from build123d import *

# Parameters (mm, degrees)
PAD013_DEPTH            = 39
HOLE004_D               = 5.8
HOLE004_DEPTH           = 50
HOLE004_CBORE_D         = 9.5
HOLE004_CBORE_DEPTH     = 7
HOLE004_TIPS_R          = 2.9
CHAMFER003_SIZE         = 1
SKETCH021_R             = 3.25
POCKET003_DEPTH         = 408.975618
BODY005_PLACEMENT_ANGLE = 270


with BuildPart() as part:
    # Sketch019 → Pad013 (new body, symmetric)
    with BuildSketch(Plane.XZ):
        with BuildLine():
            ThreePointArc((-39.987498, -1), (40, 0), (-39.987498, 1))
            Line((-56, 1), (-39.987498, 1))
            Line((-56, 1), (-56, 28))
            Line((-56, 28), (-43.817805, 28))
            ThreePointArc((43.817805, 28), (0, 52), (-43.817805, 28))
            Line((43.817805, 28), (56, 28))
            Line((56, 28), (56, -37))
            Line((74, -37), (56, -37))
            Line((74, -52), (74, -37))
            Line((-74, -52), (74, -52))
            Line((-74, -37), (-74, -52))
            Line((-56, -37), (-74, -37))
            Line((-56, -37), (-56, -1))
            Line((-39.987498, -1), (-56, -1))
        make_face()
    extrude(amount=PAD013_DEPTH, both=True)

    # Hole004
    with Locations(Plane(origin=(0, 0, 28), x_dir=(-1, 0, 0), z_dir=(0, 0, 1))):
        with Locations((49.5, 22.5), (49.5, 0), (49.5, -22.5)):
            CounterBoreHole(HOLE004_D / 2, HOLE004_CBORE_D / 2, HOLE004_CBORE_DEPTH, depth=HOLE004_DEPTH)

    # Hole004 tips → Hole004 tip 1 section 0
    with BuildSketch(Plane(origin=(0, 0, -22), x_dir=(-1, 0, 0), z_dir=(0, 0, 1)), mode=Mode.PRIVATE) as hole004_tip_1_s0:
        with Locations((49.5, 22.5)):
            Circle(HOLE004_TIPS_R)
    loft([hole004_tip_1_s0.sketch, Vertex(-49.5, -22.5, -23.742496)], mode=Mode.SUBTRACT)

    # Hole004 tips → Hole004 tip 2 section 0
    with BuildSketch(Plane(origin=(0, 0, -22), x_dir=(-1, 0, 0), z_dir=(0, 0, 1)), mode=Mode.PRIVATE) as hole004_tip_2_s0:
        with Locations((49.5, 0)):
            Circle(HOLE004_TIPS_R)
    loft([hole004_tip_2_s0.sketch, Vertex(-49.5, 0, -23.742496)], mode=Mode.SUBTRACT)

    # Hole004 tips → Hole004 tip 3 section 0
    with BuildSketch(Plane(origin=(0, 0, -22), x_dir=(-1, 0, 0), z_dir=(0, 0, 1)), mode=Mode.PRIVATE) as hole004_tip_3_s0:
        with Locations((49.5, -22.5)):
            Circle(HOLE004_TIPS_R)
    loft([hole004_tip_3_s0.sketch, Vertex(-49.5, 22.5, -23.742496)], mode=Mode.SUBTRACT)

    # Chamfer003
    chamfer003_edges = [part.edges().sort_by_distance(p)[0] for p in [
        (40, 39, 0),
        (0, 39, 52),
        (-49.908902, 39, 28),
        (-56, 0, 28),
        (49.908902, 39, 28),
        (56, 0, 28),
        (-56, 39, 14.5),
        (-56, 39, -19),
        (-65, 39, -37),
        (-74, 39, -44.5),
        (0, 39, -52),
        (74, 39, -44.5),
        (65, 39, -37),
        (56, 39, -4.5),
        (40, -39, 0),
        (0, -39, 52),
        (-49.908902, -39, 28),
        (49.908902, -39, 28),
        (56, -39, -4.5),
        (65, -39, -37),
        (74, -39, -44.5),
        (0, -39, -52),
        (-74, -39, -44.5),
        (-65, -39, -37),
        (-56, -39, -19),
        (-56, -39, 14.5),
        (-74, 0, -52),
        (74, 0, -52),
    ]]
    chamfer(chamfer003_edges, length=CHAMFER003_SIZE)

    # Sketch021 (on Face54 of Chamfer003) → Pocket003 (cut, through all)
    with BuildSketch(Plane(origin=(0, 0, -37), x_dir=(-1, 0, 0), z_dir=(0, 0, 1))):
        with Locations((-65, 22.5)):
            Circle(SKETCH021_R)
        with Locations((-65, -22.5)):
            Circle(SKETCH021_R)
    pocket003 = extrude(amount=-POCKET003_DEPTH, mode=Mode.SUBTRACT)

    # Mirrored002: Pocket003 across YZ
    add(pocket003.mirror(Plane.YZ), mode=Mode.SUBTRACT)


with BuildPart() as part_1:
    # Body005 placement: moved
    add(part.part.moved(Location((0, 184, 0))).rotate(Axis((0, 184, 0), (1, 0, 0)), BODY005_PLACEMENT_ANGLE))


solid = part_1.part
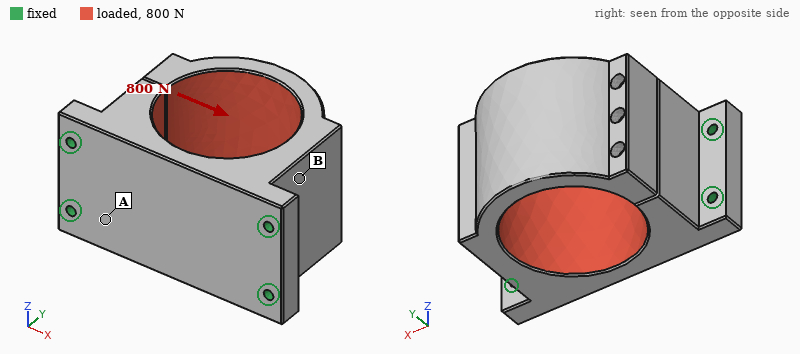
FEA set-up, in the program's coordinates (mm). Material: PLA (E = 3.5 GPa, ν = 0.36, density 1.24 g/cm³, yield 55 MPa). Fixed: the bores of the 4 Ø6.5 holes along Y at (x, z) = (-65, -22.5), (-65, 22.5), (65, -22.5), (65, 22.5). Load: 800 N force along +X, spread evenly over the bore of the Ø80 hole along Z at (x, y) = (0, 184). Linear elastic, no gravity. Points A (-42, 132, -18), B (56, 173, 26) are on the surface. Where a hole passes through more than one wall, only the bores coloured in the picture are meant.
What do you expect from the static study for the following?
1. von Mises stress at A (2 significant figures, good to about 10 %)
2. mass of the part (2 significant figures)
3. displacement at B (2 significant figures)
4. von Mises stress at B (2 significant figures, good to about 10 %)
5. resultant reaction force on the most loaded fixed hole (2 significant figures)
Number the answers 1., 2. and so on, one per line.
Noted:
1. 0.73 MPa
2. 560 g
3. 0.12 mm
4. 3.3 MPa
5. 330 N
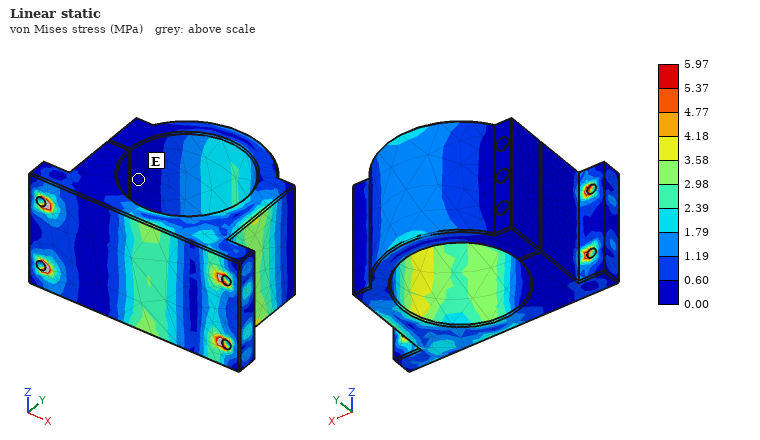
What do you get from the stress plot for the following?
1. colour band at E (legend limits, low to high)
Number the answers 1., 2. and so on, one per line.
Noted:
1. 0.00 to 0.60 MPa
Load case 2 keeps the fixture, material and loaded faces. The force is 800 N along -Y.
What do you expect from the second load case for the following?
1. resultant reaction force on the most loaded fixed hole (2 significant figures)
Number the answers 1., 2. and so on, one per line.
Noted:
1. 220 N
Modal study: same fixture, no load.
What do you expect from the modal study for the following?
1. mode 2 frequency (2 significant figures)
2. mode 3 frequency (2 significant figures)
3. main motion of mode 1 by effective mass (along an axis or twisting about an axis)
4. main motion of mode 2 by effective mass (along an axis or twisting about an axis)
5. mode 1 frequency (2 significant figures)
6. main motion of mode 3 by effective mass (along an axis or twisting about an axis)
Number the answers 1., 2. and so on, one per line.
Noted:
1. 260 Hz
2. 360 Hz
3. along Y
4. along Z
5. 170 Hz
6. along X
